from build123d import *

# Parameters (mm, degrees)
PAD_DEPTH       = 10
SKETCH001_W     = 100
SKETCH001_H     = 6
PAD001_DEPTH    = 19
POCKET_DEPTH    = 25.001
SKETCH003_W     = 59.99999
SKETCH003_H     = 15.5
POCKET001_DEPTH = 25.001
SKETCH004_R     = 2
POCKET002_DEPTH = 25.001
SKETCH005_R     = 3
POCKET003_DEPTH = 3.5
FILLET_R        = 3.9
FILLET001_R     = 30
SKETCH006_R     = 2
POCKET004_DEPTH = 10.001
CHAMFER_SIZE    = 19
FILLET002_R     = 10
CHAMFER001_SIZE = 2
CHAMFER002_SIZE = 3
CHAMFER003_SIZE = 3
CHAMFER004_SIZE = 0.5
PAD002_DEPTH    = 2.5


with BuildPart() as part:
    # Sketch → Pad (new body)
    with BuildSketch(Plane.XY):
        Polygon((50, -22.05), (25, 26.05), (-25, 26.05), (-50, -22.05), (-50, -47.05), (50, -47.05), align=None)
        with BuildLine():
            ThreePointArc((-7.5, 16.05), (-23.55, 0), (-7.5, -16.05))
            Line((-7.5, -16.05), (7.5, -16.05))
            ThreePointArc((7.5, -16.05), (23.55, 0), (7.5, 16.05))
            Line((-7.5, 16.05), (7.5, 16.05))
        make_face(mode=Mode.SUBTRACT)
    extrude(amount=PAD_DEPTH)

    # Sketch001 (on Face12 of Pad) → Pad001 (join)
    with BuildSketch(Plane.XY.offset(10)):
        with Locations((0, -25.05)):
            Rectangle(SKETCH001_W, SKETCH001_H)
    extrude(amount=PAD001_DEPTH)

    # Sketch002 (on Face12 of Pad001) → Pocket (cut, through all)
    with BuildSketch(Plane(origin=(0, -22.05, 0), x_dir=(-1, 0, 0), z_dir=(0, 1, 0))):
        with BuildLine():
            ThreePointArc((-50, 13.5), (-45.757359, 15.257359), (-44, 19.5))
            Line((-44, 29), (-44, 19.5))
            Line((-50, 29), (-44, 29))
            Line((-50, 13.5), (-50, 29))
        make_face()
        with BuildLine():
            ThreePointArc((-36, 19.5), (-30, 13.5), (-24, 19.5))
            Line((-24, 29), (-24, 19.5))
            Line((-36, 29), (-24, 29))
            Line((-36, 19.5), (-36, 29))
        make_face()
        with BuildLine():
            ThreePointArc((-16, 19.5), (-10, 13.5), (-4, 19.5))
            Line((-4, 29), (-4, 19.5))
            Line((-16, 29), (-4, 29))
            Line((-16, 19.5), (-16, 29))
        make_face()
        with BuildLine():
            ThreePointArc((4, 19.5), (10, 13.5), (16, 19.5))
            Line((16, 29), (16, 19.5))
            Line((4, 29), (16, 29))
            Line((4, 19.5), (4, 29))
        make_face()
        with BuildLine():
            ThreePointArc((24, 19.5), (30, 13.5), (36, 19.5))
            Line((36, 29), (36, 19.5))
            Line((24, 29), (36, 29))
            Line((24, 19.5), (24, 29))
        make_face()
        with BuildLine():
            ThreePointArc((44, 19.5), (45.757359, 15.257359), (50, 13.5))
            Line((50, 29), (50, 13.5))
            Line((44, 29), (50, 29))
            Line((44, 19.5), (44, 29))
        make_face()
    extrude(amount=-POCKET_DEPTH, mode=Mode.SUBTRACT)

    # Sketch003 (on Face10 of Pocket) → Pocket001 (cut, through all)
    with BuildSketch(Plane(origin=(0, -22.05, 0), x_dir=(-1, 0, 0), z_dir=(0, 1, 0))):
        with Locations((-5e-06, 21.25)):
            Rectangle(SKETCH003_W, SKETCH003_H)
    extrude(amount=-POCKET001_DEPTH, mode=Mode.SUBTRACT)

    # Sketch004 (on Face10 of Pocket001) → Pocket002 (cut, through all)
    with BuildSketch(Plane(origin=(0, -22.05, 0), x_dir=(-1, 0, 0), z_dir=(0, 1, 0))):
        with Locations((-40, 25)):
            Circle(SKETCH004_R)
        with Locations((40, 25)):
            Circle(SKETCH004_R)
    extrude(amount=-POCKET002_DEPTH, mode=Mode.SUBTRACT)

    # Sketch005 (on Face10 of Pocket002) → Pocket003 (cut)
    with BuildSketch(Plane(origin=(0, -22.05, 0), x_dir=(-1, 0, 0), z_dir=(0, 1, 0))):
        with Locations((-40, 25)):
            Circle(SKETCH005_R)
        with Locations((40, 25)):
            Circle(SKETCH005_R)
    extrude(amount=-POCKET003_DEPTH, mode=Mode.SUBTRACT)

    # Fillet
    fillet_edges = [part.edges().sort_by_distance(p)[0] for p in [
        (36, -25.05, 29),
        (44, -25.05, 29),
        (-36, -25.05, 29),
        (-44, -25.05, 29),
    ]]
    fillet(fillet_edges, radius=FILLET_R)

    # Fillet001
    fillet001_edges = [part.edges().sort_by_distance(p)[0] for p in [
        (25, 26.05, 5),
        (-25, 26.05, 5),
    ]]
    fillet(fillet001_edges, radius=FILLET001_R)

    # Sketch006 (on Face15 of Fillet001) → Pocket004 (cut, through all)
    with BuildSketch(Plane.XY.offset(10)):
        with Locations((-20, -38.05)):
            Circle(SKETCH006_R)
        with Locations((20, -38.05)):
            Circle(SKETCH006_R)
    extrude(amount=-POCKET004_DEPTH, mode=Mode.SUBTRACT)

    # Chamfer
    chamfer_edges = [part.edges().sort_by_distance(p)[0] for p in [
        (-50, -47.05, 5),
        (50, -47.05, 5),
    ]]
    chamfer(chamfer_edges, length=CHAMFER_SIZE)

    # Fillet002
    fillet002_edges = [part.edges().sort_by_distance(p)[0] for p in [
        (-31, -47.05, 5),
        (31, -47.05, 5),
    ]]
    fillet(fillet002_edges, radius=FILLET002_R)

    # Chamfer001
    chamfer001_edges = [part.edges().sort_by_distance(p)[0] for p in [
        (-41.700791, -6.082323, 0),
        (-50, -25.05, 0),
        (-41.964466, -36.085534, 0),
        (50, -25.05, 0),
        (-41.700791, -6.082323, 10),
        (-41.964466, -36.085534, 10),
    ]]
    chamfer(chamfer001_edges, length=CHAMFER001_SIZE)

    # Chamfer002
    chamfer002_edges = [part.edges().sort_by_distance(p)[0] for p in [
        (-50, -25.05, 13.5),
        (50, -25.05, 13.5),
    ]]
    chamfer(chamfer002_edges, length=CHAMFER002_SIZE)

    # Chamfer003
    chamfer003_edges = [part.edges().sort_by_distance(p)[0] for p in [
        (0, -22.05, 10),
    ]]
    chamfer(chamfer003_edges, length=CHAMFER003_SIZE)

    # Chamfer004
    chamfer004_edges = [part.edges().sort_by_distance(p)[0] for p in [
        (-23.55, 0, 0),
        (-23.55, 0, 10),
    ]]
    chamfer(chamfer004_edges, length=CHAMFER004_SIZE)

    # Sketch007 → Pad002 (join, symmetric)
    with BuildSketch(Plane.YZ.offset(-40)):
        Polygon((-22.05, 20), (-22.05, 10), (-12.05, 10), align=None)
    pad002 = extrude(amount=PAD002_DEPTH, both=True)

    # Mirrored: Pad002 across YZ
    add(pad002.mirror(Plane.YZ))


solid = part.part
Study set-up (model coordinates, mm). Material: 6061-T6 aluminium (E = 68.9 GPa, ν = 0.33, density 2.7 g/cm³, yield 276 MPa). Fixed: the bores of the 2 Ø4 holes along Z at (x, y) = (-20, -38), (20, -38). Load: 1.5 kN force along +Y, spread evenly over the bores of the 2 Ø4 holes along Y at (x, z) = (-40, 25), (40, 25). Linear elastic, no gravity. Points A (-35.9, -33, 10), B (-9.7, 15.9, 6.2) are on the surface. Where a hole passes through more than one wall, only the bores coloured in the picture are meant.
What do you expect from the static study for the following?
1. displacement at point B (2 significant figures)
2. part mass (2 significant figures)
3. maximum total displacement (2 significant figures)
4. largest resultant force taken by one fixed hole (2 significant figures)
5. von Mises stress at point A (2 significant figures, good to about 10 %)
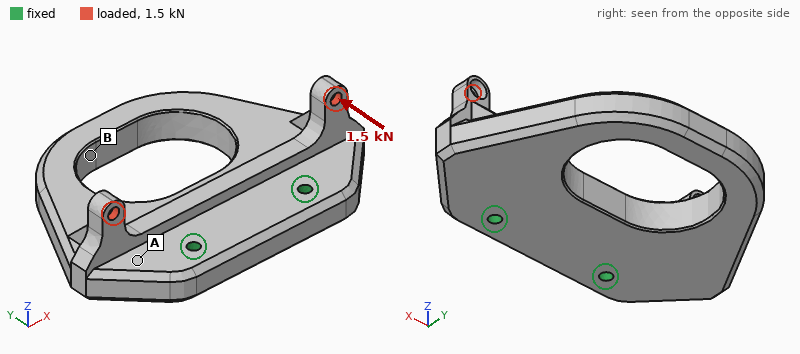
0.077 mm
130 g
0.11 mm
850 N
26 MPa
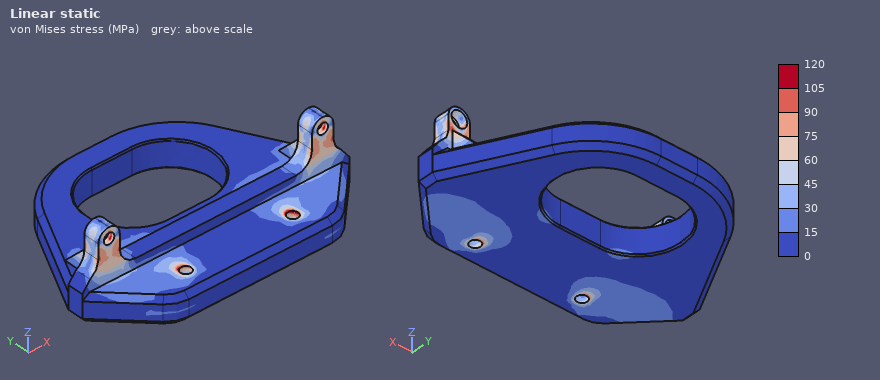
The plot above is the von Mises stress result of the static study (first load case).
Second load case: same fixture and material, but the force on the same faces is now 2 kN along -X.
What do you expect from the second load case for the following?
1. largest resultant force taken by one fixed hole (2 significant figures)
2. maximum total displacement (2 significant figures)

1.3 kN
0.11 mm
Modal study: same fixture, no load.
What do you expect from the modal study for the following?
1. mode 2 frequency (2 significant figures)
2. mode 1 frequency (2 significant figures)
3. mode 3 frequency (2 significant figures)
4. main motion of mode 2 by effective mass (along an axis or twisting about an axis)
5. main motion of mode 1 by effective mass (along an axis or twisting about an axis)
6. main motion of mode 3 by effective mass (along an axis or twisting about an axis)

3900 Hz
2200 Hz
5800 Hz
twisting about Y
along Z
along X
